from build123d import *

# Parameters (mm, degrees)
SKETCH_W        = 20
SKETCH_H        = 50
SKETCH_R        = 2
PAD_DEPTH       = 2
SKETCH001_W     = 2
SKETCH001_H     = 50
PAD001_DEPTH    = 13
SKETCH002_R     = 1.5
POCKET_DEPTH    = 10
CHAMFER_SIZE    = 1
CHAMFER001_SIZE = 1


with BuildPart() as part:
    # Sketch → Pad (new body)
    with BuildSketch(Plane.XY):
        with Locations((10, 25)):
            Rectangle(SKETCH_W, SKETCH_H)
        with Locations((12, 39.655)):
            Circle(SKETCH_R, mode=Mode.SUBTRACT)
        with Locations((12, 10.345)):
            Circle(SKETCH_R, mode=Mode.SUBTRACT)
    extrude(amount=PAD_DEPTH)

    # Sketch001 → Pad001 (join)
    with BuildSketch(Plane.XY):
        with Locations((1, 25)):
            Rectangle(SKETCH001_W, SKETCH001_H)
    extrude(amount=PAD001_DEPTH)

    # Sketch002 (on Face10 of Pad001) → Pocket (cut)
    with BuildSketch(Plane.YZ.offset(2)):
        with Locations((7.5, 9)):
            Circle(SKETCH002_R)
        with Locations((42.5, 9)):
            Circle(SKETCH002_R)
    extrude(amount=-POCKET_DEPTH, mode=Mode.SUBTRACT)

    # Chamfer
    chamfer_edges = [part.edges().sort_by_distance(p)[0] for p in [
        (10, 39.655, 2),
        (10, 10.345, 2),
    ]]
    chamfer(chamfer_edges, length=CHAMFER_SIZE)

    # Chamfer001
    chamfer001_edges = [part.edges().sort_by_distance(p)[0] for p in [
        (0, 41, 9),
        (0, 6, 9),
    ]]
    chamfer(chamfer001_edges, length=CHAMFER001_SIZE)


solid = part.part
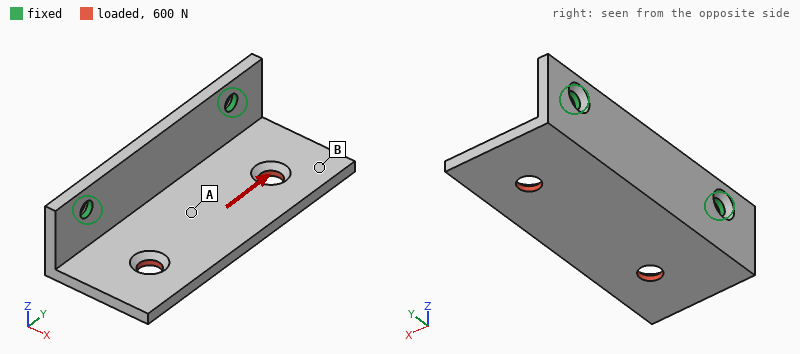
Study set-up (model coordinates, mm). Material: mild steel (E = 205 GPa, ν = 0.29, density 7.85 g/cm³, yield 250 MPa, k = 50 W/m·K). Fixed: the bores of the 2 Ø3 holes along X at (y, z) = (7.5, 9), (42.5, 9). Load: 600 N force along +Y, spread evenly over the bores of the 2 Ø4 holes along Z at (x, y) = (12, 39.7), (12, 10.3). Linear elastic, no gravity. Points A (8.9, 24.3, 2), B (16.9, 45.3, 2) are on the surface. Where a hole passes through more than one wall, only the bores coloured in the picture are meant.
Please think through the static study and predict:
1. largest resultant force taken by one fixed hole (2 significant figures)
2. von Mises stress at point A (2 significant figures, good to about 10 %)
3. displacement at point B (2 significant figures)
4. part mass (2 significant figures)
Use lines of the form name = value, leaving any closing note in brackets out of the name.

largest resultant force taken by one fixed hole = 370 N
von Mises stress at point A = 30 MPa
displacement at point B = 28 µm
part mass = 24 g
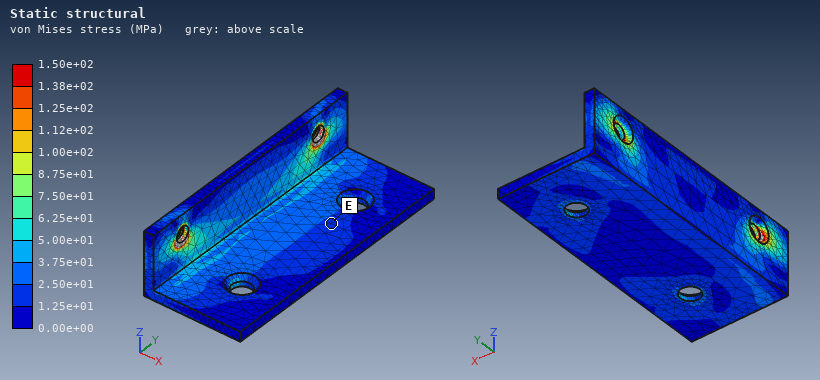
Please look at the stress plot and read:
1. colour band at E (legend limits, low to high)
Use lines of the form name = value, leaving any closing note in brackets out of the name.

colour band at E = 1.25e+01 to 2.50e+01 MPa
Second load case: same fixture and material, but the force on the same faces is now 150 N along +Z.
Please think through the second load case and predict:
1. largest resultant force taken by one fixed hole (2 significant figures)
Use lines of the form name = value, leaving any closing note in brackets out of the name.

largest resultant force taken by one fixed hole = 75 N
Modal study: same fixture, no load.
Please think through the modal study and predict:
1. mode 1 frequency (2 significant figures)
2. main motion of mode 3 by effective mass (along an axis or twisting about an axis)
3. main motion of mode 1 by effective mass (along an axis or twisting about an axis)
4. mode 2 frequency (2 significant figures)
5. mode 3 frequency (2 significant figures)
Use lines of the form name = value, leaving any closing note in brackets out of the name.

mode 1 frequency = 2300 Hz
main motion of mode 3 by effective mass = along X
main motion of mode 1 by effective mass = along Z
mode 2 frequency = 4200 Hz
mode 3 frequency = 7100 Hz
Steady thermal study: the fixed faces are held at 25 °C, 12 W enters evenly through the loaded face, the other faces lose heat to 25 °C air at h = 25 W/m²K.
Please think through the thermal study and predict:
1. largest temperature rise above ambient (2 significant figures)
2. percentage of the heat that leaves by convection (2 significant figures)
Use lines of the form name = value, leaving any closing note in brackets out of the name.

largest temperature rise above ambient = 64 K
percentage of the heat that leaves by convection = 23 %
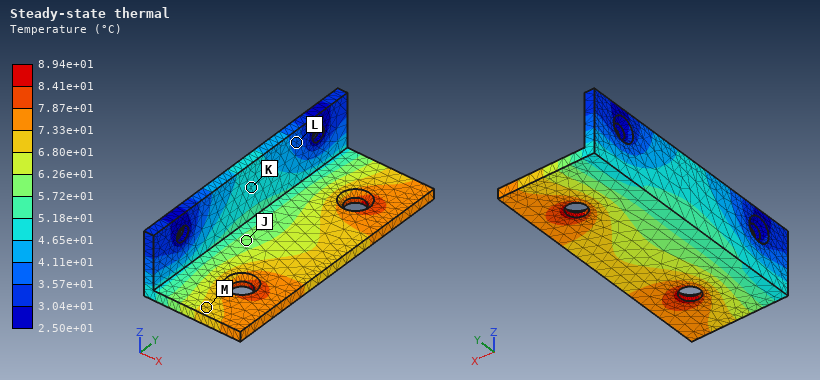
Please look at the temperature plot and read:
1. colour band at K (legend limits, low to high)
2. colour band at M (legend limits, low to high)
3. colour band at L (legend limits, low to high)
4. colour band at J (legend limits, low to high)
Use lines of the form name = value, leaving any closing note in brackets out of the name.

colour band at K = 4.65e+01 to 5.18e+01 °C
colour band at M = 6.80e+01 to 7.33e+01 °C
colour band at L = 3.57e+01 to 4.11e+01 °C
colour band at J = 5.72e+01 to 6.26e+01 °C
